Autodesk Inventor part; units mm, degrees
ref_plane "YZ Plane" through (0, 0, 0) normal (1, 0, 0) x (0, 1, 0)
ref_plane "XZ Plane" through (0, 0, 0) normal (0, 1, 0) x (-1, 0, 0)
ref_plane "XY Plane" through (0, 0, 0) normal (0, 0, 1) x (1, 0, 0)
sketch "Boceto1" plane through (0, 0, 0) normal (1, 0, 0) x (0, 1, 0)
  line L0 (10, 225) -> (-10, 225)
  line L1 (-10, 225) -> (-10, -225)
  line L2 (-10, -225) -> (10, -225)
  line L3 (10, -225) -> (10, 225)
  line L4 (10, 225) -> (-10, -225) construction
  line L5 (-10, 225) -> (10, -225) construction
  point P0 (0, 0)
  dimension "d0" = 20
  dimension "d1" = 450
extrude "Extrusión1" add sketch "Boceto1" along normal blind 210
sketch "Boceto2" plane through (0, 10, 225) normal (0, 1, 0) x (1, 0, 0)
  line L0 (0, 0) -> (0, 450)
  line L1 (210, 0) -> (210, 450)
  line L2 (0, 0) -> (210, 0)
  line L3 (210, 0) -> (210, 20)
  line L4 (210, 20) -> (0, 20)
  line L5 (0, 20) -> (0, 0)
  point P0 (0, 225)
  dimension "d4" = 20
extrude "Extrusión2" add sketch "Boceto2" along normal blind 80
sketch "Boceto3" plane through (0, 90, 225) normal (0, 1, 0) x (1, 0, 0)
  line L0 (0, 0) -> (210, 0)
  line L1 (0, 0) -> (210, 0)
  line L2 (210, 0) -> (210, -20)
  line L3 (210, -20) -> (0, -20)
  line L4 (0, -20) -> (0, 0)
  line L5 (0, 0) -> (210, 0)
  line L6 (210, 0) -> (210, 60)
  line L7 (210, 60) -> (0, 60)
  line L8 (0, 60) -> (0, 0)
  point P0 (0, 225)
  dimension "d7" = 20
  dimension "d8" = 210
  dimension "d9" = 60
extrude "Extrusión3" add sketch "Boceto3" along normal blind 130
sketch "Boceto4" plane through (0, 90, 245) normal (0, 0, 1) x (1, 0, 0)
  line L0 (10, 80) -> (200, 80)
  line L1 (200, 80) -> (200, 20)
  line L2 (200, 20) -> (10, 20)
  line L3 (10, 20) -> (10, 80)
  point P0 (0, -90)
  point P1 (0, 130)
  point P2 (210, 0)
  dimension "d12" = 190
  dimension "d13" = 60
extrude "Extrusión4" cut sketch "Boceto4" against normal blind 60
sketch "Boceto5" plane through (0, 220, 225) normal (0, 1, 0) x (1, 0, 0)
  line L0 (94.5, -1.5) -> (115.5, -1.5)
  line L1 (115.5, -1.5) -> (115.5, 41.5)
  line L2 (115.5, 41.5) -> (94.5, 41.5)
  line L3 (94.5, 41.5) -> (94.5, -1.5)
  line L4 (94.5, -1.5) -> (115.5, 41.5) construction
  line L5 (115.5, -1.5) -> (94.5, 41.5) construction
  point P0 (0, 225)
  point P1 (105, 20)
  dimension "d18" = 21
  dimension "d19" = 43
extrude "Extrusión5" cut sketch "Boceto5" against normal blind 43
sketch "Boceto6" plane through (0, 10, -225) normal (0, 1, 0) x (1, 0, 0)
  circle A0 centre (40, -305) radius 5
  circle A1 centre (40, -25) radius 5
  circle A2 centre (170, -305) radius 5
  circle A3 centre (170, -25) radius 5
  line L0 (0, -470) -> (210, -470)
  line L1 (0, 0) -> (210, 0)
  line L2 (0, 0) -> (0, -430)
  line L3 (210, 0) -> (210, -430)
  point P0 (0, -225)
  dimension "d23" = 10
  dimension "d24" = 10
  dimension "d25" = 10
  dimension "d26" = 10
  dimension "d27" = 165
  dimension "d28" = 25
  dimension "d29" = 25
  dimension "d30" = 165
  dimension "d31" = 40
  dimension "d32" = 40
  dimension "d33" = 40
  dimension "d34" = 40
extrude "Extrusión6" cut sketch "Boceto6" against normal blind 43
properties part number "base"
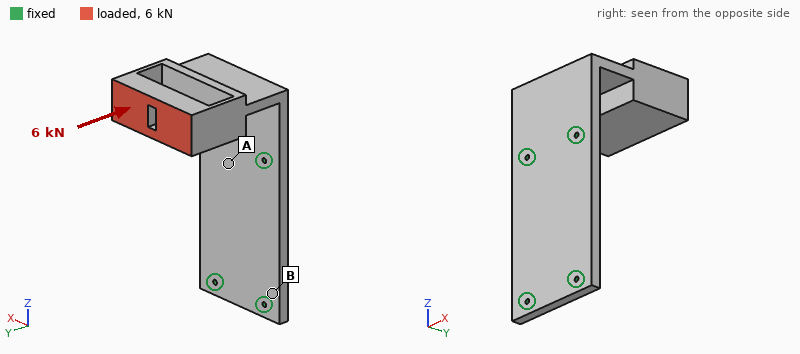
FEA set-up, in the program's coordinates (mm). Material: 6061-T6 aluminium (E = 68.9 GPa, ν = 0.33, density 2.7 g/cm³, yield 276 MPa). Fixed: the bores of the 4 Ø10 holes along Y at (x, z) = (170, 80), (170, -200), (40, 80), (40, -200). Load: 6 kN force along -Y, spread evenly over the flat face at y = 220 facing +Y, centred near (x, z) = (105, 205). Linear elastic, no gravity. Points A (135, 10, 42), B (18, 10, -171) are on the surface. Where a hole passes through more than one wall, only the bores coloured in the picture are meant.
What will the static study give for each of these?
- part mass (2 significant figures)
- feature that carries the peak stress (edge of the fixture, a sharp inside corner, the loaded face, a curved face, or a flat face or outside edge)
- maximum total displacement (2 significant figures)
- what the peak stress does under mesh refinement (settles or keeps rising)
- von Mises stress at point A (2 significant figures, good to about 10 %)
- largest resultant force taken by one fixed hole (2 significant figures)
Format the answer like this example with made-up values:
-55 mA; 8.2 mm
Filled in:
9.9 kg; edge of the fixture; 1.4 mm; keeps rising; 9.3 MPa; 3.4 kN
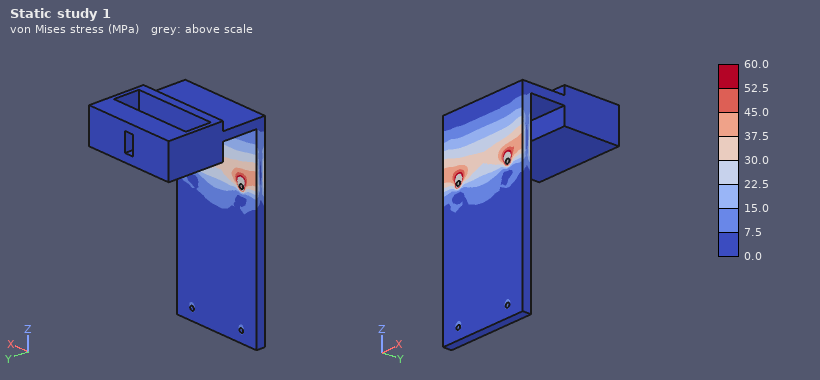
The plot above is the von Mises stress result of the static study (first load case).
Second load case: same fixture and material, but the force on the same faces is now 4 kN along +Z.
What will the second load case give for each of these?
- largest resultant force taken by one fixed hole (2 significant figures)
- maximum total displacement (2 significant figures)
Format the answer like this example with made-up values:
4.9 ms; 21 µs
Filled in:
1.9 kN; 4.1 mm
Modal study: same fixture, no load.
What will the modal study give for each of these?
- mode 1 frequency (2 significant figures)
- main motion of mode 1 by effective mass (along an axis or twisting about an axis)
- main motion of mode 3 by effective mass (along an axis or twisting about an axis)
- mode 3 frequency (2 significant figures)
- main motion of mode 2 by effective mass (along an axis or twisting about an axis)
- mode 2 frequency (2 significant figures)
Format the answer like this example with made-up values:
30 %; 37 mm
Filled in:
100 Hz; along Z; along Y; 330 Hz; along X; 190 Hz
